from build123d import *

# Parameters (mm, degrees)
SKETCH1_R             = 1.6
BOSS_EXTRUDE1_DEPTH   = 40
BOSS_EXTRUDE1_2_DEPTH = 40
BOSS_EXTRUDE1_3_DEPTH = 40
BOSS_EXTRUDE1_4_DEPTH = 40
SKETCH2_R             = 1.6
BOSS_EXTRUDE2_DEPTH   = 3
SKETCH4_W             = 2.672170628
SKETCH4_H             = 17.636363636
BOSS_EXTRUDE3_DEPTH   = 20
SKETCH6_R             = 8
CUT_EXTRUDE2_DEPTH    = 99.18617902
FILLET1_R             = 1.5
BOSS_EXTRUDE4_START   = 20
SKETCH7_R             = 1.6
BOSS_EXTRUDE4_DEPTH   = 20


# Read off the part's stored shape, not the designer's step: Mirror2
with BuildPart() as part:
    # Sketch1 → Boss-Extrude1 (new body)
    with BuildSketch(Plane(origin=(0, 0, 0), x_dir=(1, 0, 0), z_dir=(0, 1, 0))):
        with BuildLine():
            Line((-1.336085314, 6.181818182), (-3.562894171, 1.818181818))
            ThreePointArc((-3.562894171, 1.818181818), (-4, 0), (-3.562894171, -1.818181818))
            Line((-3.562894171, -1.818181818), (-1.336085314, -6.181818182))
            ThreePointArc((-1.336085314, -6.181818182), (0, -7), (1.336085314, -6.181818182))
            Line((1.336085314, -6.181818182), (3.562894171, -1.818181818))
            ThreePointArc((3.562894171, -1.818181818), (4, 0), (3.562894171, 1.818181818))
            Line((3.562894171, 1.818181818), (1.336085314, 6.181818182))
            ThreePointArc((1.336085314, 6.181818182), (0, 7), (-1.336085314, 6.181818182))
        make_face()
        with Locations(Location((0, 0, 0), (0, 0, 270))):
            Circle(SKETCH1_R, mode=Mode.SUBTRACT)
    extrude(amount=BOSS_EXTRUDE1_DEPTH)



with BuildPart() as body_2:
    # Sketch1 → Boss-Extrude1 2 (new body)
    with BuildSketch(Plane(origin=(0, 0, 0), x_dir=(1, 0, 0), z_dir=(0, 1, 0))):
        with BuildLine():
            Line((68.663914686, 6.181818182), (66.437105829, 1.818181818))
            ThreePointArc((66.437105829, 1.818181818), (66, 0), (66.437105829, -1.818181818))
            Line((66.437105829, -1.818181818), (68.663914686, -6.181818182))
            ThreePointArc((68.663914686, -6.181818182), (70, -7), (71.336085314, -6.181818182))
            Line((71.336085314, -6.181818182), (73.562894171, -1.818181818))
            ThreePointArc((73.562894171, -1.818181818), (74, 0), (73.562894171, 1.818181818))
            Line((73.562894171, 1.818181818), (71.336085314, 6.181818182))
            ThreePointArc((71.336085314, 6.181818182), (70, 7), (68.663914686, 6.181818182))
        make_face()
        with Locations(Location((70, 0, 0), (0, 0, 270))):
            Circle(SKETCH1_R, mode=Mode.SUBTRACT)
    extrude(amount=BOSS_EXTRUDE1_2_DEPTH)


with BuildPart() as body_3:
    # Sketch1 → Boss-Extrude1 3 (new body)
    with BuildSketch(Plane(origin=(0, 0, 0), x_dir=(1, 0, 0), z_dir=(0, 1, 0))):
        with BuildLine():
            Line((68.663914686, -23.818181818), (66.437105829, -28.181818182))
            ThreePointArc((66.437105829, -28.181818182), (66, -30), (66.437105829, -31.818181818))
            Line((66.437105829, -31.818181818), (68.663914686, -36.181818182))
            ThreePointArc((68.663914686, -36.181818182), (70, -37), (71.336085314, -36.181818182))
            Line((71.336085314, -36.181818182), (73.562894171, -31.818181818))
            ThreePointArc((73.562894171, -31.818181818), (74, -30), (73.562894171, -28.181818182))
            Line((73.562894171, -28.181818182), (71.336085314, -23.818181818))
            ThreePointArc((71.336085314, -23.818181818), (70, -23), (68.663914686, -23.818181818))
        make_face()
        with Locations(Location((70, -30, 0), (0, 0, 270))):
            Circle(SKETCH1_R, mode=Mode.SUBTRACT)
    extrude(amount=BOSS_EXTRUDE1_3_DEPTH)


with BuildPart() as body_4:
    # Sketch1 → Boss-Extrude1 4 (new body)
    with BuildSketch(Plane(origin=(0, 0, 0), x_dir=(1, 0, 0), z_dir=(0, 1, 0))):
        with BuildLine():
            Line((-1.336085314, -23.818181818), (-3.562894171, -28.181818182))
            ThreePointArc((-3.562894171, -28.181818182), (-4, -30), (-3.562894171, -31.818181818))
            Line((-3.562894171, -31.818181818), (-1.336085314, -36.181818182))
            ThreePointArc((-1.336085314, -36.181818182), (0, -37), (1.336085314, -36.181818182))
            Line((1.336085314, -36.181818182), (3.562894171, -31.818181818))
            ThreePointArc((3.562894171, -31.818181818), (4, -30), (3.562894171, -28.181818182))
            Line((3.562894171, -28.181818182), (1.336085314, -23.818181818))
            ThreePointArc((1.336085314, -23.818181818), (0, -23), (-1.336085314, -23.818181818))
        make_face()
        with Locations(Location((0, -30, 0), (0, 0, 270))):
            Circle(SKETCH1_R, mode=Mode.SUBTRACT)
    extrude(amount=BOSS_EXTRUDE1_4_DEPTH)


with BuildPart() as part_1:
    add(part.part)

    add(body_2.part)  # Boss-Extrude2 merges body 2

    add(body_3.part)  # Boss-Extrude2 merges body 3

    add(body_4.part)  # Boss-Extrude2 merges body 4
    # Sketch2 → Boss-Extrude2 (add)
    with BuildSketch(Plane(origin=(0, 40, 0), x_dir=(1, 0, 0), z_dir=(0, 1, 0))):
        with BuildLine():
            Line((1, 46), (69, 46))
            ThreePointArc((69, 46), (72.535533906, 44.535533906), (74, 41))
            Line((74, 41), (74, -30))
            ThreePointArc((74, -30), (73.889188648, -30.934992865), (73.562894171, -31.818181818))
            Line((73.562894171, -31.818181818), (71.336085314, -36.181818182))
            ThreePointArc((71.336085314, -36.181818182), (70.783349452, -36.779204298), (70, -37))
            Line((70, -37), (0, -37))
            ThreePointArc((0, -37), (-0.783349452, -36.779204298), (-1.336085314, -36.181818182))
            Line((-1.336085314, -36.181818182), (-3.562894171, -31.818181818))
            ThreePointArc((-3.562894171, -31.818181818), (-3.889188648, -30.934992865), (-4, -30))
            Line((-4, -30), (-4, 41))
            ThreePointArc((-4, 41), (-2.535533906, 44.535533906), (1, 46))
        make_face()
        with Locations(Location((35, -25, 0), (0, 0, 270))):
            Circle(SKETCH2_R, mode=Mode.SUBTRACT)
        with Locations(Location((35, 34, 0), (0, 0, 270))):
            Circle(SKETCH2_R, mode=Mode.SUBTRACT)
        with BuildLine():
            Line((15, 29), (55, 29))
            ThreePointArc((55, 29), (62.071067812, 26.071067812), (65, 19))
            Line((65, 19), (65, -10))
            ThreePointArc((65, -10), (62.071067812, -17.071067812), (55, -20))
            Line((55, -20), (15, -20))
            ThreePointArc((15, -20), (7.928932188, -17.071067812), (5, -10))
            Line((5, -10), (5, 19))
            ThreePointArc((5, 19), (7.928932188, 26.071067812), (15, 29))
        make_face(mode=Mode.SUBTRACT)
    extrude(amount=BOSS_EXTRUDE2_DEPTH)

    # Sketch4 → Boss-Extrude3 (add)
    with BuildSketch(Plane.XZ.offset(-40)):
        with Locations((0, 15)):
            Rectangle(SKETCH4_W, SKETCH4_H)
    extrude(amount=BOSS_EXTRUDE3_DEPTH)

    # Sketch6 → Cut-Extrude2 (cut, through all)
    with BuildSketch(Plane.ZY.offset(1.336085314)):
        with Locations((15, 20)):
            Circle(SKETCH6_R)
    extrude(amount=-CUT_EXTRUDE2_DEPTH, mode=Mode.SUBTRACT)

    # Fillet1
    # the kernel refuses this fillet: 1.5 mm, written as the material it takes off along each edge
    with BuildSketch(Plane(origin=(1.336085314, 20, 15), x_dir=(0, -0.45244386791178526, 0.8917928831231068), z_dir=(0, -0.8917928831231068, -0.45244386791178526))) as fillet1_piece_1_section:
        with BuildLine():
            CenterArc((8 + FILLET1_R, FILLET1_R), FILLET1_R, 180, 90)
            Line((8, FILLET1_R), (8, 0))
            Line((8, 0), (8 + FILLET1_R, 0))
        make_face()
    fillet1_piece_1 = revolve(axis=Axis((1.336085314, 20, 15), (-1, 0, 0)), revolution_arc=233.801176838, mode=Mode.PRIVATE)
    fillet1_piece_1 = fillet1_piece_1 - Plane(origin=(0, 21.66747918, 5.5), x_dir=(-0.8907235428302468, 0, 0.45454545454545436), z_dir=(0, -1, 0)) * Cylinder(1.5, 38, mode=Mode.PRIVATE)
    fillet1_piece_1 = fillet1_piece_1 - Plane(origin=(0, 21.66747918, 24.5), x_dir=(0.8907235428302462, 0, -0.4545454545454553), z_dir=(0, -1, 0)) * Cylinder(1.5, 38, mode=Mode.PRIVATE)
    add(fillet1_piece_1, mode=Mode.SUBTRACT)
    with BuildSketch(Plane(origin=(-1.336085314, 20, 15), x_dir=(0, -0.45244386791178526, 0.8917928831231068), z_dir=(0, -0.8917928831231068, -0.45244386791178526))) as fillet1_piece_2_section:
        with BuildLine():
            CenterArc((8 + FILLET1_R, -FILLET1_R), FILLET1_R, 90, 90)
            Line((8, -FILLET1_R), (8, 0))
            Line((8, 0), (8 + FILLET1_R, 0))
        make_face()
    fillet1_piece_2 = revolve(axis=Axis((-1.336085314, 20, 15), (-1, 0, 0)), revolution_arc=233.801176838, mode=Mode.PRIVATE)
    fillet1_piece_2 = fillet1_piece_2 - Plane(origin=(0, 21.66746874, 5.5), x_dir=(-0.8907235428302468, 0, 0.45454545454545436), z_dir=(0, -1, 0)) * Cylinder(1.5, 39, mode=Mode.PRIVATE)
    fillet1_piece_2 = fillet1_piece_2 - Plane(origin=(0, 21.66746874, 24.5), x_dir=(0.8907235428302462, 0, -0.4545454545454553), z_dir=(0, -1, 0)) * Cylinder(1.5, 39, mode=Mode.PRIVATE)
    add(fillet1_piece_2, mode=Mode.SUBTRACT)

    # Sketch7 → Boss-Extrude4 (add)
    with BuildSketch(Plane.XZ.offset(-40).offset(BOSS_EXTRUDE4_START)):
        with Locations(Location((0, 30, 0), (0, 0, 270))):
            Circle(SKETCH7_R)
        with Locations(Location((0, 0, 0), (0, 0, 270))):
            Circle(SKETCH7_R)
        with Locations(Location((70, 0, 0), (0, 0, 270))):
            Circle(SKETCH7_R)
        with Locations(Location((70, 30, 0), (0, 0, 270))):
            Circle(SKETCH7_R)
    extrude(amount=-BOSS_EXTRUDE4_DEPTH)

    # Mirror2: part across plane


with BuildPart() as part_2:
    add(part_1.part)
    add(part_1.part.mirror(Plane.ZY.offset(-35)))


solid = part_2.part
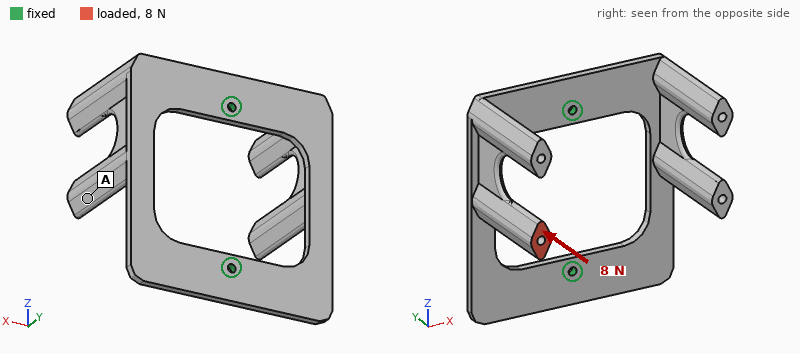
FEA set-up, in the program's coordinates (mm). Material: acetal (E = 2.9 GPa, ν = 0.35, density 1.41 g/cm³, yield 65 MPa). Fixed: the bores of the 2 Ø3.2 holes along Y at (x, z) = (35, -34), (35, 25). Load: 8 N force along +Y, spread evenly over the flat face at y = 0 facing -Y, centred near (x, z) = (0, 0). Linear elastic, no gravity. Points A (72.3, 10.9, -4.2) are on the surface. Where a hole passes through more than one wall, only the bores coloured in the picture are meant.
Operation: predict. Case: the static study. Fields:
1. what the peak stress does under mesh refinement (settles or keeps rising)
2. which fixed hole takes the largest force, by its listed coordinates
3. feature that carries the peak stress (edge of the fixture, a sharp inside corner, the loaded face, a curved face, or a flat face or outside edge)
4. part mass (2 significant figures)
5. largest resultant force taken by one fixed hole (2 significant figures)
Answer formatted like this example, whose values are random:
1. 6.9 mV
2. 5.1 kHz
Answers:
1. keeps rising
2. (35, 25)
3. edge of the fixture
4. 33 g
5. 4.3 N
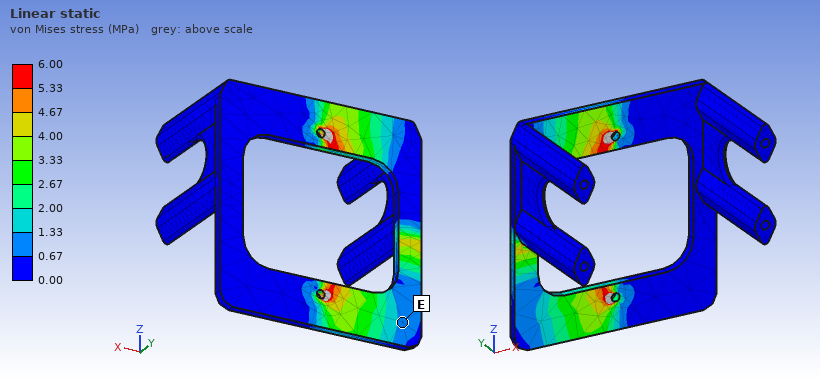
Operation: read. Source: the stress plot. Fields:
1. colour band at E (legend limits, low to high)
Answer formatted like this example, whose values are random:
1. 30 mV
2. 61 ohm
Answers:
1. 0.67 to 1.33 MPa
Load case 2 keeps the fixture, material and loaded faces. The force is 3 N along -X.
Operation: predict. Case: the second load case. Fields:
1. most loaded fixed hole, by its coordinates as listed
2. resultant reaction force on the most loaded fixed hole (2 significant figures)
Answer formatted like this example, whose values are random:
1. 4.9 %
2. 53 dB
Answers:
1. (35, 25)
2. 2.0 N
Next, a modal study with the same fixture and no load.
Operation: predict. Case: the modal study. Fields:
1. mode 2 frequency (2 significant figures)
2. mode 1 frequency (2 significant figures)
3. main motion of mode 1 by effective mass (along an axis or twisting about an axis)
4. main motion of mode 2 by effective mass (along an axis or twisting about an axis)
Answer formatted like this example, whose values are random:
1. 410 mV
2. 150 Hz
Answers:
1. 130 Hz
2. 120 Hz
3. along X
4. along Y
